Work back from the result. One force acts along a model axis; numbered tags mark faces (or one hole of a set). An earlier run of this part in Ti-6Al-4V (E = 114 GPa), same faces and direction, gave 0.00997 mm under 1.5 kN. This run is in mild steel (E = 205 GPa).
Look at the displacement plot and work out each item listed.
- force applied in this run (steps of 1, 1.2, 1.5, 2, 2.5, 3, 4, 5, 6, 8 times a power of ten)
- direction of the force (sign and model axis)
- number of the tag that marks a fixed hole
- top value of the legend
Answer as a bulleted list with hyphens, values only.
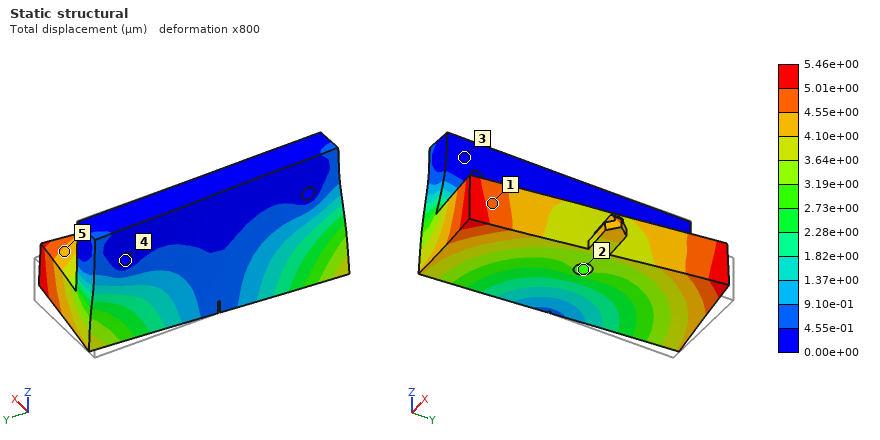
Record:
- 1.5 kN
- -Y
- 4
- 5.46e+00 µm
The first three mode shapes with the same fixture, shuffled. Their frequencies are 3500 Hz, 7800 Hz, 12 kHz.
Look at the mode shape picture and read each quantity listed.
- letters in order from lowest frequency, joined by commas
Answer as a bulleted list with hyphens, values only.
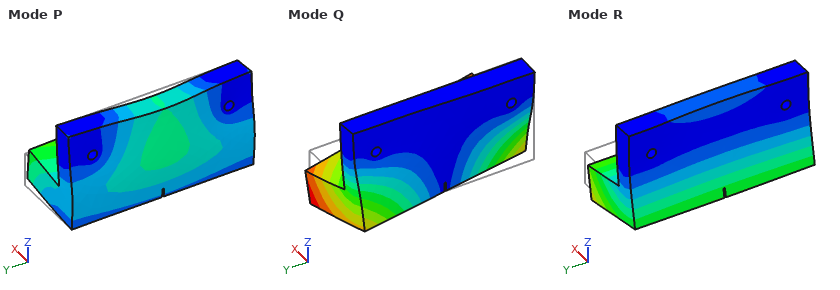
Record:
- R, Q, P
